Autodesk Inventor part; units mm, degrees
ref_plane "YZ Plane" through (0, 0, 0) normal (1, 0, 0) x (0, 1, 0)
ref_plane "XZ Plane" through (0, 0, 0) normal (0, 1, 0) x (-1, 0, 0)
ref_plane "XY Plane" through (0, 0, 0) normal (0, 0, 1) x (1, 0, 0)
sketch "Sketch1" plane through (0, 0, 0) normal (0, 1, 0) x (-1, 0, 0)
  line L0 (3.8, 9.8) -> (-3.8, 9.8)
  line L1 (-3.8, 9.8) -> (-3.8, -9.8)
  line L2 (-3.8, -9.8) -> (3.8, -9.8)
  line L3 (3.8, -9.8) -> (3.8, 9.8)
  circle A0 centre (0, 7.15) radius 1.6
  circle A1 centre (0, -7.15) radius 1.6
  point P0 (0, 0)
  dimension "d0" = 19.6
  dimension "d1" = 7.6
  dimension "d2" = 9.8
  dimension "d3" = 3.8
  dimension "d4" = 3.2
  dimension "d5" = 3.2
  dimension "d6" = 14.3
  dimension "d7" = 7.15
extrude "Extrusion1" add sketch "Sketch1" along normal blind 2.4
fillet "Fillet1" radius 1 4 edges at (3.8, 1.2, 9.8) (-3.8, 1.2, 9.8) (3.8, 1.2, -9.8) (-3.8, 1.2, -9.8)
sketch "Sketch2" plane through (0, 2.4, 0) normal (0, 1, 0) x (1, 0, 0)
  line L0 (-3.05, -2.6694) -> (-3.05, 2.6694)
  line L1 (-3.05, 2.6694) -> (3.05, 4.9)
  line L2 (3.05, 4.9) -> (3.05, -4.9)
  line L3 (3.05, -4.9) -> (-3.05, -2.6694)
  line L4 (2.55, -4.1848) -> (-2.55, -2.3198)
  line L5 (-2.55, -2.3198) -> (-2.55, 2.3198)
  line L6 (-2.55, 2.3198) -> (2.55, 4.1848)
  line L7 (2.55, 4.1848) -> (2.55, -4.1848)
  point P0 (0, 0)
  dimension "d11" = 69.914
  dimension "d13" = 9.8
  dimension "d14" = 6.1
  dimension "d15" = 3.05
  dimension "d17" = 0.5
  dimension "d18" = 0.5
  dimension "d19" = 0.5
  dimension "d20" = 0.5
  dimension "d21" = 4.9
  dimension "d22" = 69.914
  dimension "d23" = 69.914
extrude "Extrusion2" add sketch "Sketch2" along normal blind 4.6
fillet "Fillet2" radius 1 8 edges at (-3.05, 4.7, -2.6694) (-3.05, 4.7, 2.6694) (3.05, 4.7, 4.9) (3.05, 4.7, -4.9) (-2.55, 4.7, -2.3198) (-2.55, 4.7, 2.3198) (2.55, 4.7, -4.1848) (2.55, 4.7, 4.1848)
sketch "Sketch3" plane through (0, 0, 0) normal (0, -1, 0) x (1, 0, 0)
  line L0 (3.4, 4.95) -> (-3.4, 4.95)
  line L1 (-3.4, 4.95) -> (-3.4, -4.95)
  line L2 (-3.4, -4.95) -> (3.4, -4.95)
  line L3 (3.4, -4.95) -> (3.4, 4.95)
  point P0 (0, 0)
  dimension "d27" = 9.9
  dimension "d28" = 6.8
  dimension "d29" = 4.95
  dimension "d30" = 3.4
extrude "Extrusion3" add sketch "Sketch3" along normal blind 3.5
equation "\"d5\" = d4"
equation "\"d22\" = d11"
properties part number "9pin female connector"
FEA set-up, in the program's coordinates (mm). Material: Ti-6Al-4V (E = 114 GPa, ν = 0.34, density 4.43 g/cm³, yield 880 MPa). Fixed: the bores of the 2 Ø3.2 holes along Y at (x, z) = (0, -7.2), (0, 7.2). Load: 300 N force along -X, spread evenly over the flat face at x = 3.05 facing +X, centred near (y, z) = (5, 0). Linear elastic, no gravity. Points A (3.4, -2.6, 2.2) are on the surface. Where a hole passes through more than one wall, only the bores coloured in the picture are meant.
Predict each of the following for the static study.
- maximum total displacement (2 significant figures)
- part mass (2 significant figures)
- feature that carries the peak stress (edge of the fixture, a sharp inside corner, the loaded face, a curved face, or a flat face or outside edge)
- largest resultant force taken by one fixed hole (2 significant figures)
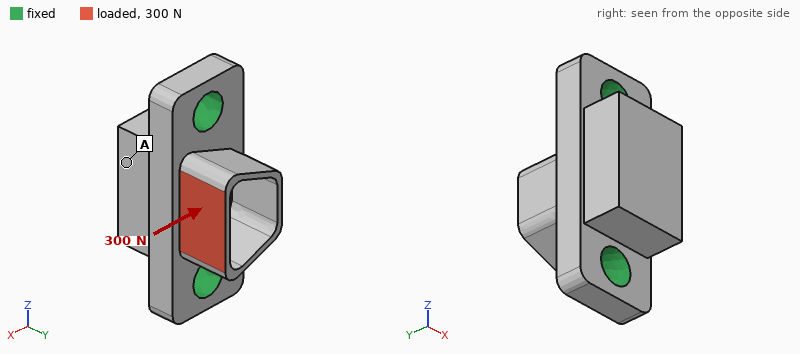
89 µm
2.7 g
the loaded face
160 N
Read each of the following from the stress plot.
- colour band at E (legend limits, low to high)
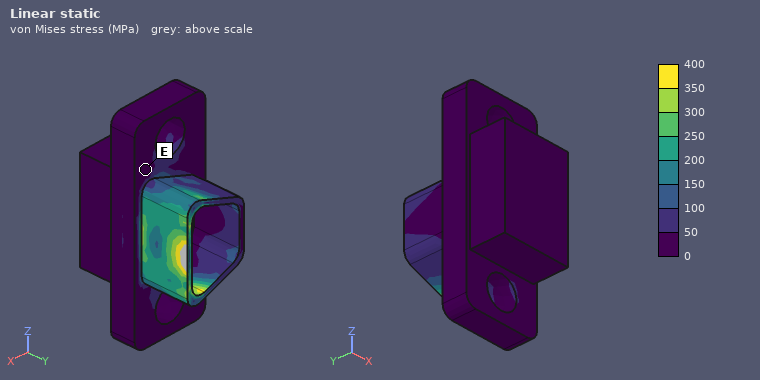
0 to 50 MPa
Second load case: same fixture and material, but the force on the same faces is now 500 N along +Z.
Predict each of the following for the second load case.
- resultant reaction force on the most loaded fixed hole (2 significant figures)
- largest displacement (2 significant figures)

310 N
11 µm
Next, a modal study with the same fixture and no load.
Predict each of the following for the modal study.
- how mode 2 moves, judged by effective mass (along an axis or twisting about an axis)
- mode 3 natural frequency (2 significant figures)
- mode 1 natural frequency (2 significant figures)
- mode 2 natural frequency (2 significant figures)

along X
63 kHz
39 kHz
47 kHz
